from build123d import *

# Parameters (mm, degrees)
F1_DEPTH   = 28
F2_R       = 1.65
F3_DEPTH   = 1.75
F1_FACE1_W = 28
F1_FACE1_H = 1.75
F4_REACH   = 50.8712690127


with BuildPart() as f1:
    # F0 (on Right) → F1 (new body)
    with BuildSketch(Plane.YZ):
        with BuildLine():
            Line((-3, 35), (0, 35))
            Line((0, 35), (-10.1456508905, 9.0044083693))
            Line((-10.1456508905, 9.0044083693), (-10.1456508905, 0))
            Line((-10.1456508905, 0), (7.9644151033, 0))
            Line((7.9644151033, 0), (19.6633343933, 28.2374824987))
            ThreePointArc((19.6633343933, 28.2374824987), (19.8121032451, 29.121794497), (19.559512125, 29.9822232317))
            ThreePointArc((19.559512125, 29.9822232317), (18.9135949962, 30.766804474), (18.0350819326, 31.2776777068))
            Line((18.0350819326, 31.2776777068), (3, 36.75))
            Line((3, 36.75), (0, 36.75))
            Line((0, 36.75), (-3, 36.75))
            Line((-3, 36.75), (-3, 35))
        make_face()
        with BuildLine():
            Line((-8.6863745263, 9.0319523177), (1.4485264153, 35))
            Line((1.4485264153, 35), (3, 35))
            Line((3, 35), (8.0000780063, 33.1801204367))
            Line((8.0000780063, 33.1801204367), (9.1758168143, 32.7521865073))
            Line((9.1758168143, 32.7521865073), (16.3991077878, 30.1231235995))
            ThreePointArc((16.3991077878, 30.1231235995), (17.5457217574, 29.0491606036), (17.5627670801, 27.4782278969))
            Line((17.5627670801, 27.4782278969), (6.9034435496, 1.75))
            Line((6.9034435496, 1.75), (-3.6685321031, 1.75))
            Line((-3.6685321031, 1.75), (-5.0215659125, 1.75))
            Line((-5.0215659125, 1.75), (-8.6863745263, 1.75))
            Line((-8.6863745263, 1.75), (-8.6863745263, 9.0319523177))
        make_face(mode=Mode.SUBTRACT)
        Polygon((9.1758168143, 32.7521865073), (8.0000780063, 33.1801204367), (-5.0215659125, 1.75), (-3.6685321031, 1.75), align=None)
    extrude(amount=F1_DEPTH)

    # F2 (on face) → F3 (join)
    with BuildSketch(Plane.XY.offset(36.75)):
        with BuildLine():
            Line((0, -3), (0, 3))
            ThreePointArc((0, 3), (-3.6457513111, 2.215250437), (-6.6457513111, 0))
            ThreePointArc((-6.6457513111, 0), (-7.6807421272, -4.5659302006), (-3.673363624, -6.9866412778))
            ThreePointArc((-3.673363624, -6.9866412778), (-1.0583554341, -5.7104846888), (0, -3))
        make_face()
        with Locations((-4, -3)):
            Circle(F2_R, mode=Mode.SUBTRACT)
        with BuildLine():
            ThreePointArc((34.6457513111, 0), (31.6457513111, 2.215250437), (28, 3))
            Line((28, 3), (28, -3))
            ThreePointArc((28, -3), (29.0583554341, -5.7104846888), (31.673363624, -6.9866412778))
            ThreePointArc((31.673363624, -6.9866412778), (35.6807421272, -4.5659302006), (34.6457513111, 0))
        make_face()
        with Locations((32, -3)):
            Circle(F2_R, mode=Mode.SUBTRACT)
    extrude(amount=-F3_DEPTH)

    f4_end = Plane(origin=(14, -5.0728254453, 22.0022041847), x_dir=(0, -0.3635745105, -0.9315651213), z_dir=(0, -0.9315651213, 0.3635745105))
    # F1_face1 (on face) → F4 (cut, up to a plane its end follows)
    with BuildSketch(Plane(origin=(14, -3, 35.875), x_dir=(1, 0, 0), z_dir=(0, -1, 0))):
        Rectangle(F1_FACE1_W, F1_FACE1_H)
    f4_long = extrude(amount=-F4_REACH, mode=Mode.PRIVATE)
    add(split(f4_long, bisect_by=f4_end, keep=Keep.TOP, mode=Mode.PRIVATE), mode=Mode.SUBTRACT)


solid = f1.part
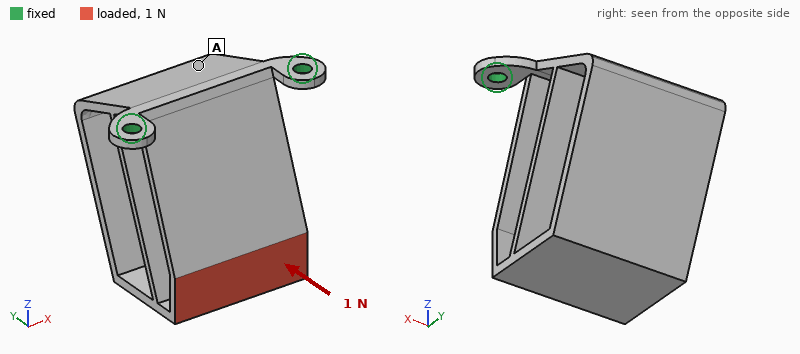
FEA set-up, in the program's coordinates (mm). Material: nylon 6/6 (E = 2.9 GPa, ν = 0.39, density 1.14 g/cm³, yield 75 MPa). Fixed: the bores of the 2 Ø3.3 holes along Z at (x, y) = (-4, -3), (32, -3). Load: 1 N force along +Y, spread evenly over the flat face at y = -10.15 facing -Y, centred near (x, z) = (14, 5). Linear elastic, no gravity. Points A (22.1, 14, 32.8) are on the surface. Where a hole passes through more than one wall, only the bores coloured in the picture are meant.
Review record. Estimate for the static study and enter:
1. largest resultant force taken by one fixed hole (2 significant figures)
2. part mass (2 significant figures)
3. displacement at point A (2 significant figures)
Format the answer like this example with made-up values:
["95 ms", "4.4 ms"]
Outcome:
["1.2 N", "6.8 g", "0.26 mm"]
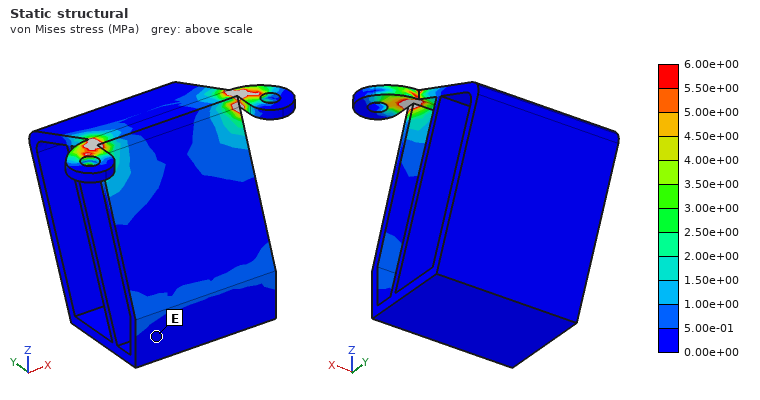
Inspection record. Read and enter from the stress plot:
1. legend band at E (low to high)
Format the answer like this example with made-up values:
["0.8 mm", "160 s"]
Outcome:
["0.00e+00 to 5.00e-01 MPa"]
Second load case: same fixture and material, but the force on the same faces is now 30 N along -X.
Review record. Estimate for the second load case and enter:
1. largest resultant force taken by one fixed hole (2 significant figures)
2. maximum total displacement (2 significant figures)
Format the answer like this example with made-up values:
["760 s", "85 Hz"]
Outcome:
["36 N", "0.40 mm"]
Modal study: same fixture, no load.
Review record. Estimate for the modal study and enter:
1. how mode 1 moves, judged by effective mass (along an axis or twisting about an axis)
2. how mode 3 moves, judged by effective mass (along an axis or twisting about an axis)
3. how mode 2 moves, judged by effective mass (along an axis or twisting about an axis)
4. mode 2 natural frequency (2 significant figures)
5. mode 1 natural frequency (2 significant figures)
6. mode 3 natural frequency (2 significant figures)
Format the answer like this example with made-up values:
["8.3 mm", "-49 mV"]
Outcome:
["along Y", "along Z", "along X", "590 Hz", "100 Hz", "740 Hz"]
